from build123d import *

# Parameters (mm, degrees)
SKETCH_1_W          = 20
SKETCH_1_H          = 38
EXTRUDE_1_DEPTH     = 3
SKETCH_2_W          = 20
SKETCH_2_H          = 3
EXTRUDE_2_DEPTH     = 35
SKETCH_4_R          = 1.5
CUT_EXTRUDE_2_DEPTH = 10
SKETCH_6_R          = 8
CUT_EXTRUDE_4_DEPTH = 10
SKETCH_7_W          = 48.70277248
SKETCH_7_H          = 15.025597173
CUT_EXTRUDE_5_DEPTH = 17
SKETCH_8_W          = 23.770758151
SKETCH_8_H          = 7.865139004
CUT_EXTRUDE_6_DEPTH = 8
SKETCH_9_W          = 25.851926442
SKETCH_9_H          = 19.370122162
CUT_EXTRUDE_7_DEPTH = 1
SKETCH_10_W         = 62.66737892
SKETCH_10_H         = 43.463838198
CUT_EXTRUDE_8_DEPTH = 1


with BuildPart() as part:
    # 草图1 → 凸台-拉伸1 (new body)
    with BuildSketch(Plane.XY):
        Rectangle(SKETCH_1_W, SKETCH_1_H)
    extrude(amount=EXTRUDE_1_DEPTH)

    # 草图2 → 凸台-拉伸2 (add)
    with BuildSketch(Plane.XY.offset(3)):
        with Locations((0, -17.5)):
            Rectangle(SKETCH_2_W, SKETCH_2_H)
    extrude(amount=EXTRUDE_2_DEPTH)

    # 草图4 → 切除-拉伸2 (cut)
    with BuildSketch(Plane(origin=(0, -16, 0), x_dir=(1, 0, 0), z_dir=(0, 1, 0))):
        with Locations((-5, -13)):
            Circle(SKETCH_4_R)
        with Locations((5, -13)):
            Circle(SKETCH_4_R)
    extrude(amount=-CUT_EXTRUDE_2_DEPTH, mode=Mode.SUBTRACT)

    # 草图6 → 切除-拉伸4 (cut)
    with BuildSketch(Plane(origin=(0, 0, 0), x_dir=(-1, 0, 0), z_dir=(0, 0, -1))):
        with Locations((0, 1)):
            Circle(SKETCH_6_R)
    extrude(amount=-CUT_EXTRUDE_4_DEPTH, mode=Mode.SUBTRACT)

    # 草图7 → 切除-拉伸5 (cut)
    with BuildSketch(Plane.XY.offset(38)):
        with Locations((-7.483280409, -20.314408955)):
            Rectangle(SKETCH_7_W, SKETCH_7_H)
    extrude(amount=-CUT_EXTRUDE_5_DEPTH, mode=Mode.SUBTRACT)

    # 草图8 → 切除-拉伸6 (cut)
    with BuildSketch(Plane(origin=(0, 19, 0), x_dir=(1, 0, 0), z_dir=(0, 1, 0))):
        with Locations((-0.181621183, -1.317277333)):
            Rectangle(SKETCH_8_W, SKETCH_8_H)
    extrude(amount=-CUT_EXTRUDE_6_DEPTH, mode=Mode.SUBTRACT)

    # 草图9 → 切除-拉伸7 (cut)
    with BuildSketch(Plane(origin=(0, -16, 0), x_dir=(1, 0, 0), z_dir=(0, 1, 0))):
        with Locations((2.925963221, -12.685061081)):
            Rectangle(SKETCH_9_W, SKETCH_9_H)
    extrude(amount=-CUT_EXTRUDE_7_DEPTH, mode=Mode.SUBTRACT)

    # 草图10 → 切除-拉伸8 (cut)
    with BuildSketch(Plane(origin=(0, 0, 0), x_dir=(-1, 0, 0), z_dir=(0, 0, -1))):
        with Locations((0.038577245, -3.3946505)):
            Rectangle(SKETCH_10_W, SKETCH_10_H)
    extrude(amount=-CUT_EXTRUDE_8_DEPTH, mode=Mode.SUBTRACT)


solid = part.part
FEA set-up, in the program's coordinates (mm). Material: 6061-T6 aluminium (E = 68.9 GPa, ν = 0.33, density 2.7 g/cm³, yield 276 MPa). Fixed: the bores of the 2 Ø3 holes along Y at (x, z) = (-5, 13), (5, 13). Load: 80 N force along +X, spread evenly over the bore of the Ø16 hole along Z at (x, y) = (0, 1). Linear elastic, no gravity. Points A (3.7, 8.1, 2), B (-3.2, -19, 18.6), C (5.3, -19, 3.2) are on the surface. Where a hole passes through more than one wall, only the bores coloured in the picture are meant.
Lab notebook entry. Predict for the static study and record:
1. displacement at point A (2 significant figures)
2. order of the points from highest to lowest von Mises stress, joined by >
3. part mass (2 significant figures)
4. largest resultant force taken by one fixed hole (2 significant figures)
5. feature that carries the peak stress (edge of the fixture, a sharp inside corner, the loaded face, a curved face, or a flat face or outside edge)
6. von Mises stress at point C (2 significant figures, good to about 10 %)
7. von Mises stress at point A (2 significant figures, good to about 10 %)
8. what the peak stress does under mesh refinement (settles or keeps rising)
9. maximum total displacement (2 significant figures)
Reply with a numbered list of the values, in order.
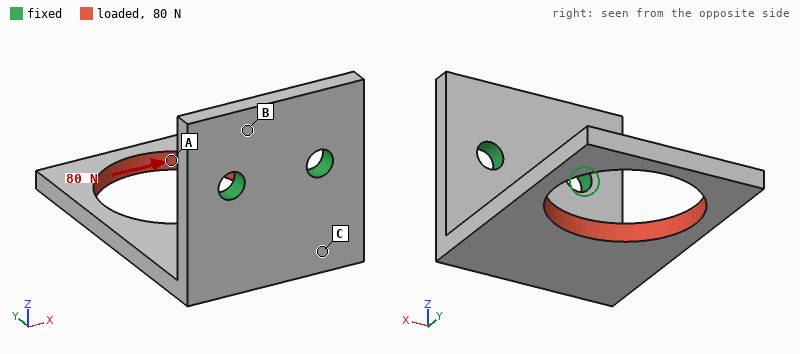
1. 0.16 mm
2. C > A > B
3. 4.0 g
4. 140 N
5. edge of the fixture
6. 48 MPa
7. 21 MPa
8. keeps rising
9. 0.19 mm
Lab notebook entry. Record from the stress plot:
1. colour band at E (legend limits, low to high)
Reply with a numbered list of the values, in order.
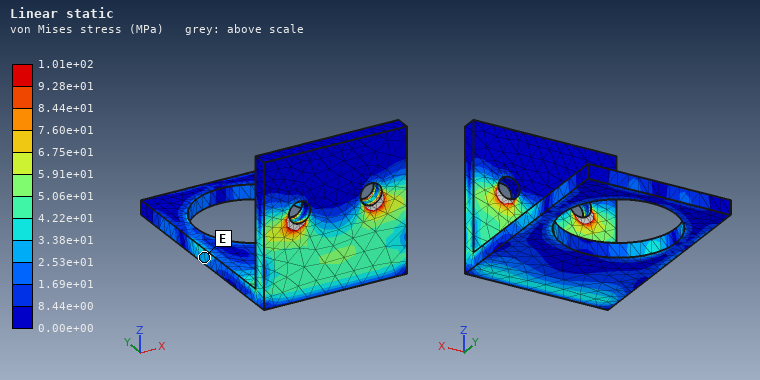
1. 2.53e+01 to 3.38e+01 MPa
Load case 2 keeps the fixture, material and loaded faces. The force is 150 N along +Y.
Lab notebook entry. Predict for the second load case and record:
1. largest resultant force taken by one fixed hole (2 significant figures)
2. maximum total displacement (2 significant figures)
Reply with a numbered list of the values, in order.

1. 75 N
2. 0.25 mm
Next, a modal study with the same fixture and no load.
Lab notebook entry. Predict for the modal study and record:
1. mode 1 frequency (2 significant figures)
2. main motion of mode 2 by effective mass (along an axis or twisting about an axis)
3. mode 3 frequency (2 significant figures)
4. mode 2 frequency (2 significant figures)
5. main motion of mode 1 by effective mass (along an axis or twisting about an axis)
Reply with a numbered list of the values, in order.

1. 1600 Hz
2. along X
3. 5000 Hz
4. 3400 Hz
5. along Z
